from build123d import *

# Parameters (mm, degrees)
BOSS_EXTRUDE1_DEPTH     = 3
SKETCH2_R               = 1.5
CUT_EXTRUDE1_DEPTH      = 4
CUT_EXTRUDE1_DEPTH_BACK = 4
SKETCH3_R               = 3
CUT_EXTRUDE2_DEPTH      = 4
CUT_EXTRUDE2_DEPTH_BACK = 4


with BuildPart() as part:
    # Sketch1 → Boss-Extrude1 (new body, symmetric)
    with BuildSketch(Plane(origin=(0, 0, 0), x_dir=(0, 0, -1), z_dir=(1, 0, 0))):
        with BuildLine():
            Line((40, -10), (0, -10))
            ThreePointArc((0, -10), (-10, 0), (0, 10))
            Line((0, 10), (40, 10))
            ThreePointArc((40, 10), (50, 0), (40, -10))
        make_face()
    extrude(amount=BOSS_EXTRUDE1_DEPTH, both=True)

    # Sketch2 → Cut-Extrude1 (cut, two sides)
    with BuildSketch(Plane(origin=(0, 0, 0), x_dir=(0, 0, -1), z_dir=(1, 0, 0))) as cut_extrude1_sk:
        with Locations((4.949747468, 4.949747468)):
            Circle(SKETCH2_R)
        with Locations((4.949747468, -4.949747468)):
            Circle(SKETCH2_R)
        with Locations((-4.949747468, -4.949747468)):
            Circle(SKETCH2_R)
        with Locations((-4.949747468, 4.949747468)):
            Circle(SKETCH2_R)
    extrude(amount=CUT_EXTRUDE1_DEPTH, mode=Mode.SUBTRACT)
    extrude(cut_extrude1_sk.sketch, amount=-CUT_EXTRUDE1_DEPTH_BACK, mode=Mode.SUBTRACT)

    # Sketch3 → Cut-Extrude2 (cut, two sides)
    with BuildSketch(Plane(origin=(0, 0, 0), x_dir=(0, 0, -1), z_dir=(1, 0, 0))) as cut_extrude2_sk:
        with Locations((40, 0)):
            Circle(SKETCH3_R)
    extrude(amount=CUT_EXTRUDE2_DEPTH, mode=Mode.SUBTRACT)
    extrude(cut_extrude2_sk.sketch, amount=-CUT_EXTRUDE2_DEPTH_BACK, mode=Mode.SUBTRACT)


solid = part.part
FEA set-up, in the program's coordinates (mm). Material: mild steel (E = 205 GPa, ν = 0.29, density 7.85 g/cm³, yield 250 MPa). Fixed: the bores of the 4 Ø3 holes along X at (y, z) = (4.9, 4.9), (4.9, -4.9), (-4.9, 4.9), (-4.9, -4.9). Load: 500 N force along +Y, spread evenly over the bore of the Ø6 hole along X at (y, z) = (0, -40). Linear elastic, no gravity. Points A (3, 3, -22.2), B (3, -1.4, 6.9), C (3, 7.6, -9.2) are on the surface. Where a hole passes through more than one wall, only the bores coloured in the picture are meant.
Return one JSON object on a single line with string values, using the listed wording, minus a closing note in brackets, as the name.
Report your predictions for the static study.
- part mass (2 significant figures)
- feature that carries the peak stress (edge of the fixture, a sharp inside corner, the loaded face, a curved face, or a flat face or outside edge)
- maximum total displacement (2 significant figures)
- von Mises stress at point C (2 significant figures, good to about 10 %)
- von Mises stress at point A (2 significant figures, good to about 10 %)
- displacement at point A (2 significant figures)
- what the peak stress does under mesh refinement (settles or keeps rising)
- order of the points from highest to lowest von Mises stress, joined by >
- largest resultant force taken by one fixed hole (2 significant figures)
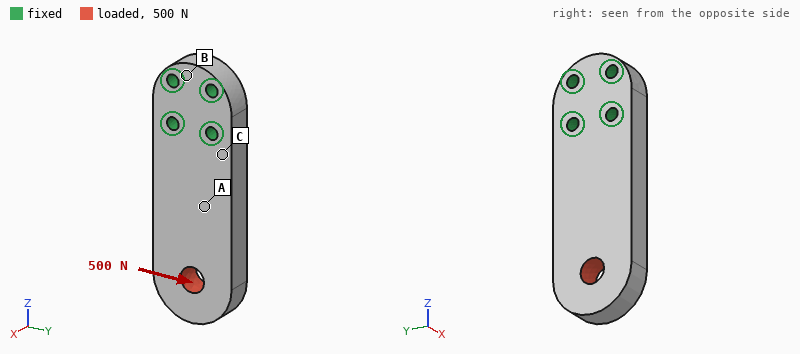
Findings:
{"part mass": "50 g", "feature that carries the peak stress": "edge of the fixture", "maximum total displacement": "16 µm", "von Mises stress at point C": "28 MPa", "von Mises stress at point A": "12 MPa", "displacement at point A": "4.3 µm", "what the peak stress does under mesh refinement": "keeps rising", "order of the points from highest to lowest von Mises stress, joined by >": "C > A > B", "largest resultant force taken by one fixed hole": "1.2 kN"}
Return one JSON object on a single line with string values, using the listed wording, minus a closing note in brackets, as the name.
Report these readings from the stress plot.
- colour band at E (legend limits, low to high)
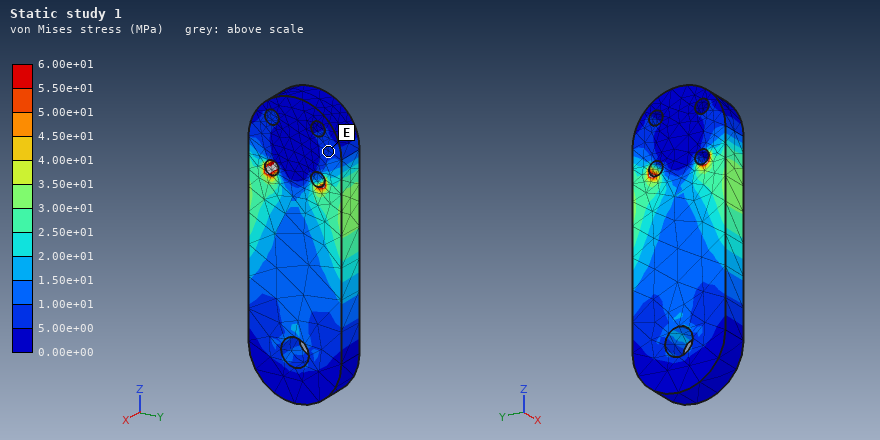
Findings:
{"colour band at E": "5.00e+00 to 1.00e+01 MPa"}
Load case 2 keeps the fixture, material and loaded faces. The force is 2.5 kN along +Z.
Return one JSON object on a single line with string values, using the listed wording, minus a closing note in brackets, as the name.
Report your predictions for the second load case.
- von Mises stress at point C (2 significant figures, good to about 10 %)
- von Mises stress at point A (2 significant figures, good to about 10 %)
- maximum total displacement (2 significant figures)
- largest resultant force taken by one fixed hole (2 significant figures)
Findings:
{"von Mises stress at point C": "19 MPa", "von Mises stress at point A": "21 MPa", "maximum total displacement": "4.7 µm", "largest resultant force taken by one fixed hole": "1.1 kN"}
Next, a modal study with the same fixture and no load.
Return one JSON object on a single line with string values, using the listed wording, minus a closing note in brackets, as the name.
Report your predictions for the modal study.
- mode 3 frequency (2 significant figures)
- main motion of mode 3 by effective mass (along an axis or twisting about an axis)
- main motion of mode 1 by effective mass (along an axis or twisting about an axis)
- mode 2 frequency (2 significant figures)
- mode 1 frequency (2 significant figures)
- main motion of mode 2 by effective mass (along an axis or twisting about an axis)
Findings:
{"mode 3 frequency": "11 kHz", "main motion of mode 3 by effective mass": "twisting about Z", "main motion of mode 1 by effective mass": "along X", "mode 2 frequency": "7600 Hz", "mode 1 frequency": "2800 Hz", "main motion of mode 2 by effective mass": "along Y"}
